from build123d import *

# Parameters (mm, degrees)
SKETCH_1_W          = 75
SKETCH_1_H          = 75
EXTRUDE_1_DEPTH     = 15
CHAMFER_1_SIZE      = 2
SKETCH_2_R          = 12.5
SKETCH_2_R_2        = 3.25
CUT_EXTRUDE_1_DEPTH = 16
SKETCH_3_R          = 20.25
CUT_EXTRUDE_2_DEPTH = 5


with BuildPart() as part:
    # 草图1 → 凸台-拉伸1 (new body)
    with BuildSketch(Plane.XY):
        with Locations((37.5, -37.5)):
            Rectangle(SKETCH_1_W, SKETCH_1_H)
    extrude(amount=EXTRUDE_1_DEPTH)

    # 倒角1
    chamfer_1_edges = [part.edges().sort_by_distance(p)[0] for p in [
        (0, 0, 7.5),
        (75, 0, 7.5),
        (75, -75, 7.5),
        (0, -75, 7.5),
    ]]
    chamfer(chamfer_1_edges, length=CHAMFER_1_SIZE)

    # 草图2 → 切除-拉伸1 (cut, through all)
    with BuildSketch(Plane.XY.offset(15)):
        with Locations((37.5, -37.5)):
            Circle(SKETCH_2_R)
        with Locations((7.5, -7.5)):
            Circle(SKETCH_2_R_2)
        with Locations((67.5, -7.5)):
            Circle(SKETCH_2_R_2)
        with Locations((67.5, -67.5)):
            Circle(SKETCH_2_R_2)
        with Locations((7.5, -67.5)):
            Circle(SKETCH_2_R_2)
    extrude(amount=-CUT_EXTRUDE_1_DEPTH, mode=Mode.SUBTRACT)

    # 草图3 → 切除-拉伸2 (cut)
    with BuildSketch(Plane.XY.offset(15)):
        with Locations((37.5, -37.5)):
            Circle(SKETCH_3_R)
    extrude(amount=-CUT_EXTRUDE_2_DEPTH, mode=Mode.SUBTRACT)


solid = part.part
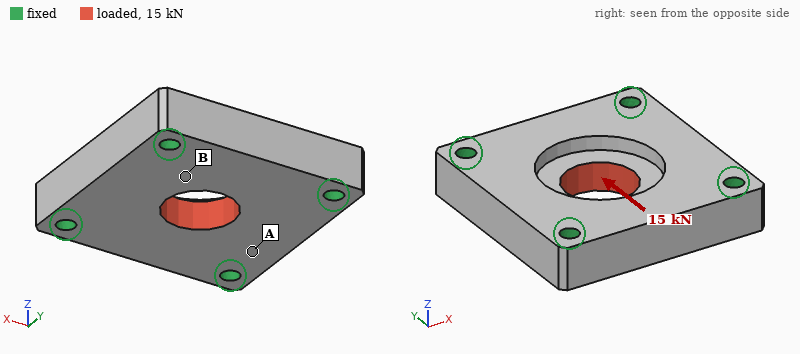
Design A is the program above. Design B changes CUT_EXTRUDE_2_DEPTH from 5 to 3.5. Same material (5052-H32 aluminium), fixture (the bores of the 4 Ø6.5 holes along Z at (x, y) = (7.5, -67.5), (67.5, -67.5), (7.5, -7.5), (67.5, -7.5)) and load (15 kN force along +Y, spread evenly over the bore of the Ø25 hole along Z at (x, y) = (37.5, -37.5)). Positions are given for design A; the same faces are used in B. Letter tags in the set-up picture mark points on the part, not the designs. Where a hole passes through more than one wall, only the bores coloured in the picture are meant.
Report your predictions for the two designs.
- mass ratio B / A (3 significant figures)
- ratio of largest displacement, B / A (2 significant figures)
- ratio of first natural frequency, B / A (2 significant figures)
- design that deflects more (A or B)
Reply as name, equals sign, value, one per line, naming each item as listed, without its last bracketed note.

mass ratio B / A = 1.02
ratio of largest displacement, B / A = 0.91
ratio of first natural frequency, B / A = 0.98
design that deflects more = A
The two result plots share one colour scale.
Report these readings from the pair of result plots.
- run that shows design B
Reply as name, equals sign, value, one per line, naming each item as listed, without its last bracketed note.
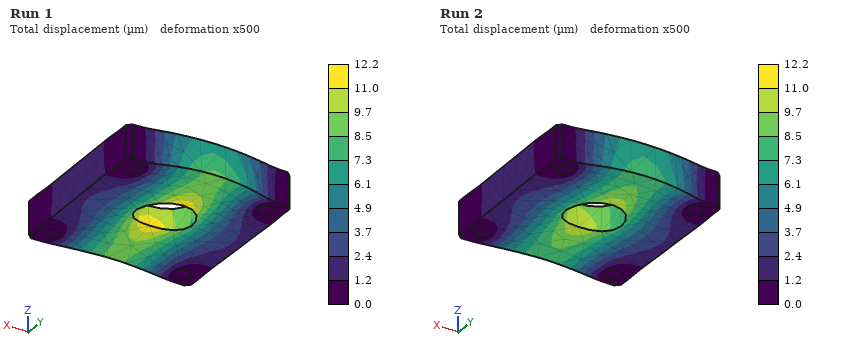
run that shows design B = Run 2
